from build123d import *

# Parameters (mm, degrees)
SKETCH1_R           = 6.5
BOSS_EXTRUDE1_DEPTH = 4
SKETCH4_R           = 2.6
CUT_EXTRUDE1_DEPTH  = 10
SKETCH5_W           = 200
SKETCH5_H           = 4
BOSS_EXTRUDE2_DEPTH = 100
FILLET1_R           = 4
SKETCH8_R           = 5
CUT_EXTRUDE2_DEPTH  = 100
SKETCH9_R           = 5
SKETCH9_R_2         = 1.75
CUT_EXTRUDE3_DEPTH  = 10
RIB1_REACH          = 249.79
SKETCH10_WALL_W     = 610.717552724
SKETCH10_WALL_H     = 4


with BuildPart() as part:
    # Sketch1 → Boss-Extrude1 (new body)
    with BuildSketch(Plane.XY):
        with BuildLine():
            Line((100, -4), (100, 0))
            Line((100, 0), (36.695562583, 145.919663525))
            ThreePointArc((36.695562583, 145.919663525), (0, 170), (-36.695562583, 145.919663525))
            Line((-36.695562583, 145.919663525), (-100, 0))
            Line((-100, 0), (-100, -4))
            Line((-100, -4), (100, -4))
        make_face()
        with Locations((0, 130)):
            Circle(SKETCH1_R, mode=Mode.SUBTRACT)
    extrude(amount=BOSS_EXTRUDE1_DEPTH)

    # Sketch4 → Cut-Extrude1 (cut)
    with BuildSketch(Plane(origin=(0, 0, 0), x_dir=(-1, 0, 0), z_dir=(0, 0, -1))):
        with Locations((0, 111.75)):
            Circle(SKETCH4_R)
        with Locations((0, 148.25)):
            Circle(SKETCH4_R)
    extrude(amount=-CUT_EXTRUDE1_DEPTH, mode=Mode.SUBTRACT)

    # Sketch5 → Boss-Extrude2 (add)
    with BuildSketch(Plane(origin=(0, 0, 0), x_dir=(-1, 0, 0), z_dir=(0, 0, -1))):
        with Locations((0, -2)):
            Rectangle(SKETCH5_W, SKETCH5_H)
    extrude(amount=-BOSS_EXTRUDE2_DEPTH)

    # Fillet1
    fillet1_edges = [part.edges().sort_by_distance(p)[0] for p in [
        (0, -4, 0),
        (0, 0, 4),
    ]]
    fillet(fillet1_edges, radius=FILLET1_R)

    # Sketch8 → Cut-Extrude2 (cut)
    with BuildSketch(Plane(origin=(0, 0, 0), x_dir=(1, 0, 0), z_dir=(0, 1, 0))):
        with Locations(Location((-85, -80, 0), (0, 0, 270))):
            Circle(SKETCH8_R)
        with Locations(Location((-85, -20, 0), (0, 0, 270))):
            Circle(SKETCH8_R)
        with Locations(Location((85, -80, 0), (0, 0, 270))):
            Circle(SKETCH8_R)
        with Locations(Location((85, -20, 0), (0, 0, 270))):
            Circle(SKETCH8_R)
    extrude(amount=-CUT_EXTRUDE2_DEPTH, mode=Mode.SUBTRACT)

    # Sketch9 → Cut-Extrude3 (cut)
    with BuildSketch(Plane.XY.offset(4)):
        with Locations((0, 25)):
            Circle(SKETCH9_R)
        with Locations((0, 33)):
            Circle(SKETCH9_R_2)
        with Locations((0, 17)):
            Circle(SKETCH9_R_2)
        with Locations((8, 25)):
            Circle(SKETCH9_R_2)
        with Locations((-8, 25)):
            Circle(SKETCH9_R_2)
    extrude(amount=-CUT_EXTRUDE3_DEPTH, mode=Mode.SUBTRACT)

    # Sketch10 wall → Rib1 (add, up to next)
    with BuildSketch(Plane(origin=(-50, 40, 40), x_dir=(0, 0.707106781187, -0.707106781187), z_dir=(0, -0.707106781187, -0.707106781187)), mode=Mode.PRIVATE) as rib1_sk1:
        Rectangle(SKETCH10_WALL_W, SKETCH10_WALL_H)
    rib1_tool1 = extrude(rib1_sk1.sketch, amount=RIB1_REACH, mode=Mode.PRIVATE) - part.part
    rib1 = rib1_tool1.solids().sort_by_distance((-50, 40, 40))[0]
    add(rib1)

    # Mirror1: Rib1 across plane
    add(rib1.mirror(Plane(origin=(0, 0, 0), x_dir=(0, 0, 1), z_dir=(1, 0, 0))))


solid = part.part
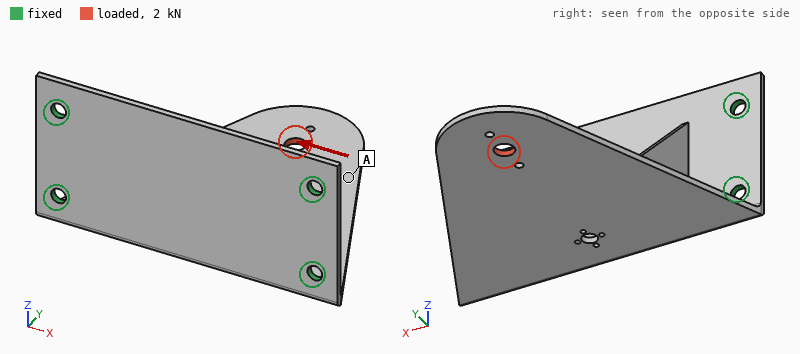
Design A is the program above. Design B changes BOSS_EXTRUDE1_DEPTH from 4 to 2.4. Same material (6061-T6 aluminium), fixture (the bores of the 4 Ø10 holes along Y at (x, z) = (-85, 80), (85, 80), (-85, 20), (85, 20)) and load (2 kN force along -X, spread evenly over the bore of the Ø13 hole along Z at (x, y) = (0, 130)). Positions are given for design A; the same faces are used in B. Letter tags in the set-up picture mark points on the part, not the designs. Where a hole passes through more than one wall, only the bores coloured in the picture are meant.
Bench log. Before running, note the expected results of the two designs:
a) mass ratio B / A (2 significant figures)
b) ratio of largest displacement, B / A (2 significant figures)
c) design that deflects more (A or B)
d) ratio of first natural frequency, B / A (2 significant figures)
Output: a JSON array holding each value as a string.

["0.82", "1.4", "B", "0.72"]
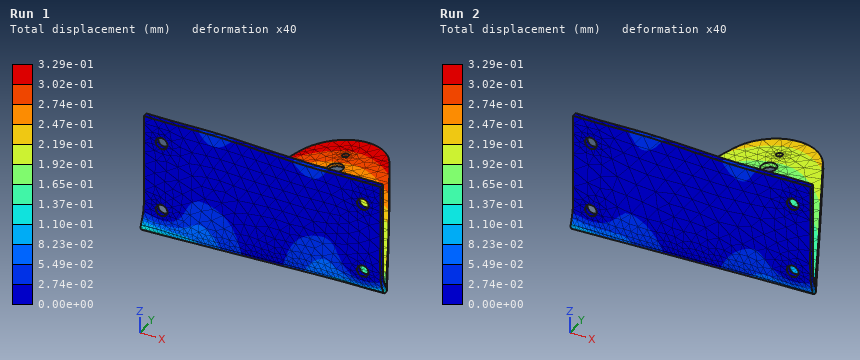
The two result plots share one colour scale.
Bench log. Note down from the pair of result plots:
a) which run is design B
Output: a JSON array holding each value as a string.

["Run 1"]
